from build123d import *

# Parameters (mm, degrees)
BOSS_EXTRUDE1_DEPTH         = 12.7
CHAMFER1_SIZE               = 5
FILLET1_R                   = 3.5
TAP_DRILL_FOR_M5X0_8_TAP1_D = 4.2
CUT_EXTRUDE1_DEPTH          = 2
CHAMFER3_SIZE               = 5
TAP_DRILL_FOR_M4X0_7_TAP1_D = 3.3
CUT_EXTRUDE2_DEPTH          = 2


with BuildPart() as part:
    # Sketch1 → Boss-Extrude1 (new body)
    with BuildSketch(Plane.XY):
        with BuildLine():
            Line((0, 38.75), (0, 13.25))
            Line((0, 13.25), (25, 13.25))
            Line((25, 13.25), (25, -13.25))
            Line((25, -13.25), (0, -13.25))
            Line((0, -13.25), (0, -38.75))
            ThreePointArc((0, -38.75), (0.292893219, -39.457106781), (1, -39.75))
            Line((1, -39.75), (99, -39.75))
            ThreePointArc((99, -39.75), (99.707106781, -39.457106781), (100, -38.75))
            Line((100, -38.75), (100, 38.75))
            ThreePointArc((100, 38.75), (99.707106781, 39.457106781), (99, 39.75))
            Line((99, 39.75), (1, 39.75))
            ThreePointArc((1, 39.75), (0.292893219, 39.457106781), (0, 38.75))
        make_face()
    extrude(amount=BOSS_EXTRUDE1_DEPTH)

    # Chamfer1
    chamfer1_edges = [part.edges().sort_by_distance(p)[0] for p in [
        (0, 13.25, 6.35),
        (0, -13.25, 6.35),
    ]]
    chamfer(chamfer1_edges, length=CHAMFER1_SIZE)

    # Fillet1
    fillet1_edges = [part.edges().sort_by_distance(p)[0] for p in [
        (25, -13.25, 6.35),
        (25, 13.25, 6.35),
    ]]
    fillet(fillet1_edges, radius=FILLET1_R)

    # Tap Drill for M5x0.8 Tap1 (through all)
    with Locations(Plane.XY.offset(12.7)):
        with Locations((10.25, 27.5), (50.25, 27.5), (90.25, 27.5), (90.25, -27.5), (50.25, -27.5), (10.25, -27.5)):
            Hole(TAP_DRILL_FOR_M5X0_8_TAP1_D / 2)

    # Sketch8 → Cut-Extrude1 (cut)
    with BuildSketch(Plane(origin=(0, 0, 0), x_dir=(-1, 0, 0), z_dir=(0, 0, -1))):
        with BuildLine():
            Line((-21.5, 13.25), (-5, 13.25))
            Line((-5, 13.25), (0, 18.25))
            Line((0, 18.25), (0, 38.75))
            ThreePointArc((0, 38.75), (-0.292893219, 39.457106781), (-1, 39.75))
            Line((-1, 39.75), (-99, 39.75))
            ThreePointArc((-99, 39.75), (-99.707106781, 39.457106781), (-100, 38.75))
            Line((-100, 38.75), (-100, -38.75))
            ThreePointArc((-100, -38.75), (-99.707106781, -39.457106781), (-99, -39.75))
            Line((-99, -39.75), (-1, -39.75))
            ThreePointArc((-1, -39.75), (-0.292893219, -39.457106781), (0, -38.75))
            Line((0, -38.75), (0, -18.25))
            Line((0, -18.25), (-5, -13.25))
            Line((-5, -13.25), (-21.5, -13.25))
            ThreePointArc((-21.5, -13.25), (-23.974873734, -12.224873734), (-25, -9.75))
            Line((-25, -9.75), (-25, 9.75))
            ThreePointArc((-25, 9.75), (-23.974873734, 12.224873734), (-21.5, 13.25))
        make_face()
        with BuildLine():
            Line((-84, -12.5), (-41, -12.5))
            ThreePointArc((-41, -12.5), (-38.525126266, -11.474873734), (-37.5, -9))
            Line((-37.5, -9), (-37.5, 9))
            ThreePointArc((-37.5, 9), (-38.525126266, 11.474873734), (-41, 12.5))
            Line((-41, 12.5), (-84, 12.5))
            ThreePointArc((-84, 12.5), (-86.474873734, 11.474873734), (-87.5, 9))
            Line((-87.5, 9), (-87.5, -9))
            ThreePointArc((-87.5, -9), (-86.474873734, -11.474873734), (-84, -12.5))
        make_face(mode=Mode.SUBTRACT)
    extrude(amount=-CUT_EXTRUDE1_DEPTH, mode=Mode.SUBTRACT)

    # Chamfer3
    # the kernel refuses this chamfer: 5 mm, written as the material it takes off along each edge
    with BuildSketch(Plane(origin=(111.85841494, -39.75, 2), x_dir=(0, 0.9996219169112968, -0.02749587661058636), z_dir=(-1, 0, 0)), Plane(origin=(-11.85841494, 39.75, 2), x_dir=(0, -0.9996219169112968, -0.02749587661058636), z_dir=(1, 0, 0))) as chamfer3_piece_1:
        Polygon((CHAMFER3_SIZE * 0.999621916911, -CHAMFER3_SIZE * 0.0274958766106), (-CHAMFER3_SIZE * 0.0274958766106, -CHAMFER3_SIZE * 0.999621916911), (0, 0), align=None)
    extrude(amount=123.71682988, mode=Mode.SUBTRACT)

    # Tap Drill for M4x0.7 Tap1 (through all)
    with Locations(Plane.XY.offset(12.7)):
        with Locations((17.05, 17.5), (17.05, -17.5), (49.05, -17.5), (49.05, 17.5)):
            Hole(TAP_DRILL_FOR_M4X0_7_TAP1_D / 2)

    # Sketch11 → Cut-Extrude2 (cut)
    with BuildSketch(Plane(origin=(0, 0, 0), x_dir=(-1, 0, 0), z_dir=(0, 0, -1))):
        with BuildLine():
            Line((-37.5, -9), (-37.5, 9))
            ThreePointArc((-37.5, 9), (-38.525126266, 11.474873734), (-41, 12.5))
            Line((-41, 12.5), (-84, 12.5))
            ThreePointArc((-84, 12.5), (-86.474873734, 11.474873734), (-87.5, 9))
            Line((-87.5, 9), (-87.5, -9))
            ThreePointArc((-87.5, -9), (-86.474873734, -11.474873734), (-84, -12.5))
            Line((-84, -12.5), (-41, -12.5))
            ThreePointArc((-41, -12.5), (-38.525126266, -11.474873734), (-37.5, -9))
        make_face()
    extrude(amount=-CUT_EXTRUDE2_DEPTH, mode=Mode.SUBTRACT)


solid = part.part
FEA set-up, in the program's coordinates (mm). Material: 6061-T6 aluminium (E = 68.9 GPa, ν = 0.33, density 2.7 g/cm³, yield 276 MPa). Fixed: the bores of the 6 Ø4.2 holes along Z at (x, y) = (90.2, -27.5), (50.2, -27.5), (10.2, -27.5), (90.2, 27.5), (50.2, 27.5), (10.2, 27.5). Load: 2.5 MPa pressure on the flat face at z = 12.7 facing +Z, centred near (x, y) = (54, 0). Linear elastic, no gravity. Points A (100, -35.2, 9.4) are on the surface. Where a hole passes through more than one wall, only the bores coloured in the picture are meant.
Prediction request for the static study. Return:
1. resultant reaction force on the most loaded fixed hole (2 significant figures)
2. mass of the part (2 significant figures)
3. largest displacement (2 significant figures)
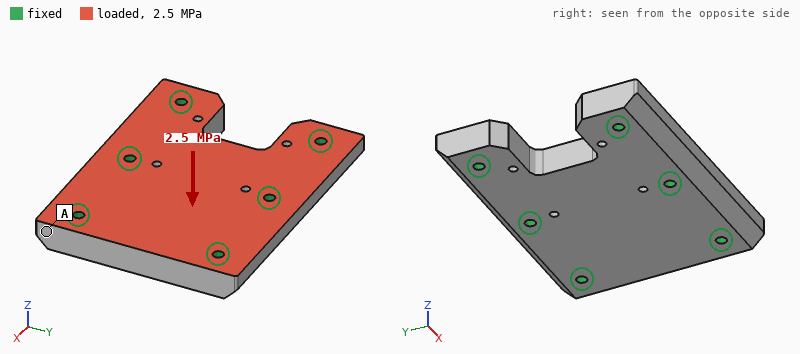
3.9 kN
200 g
20 µm
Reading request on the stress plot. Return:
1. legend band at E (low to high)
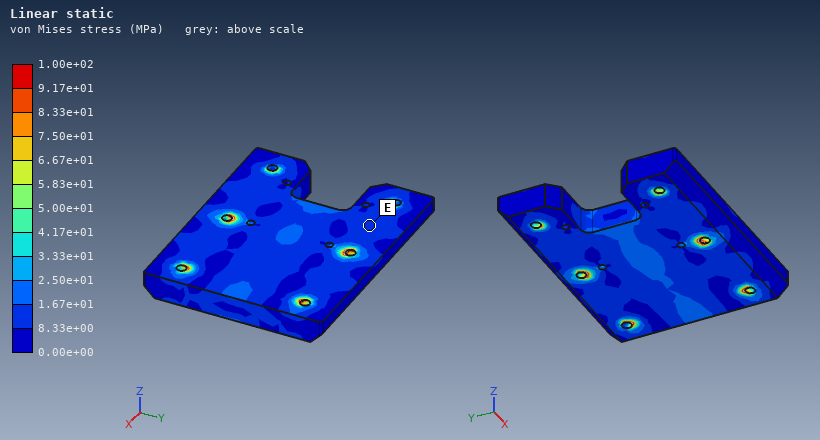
8.33e+00 to 1.67e+01 MPa
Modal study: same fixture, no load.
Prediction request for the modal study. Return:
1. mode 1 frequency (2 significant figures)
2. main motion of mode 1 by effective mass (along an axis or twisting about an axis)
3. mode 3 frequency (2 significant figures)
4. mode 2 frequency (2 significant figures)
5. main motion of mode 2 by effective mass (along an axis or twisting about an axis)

12 kHz
along Z
19 kHz
14 kHz
twisting about Y
